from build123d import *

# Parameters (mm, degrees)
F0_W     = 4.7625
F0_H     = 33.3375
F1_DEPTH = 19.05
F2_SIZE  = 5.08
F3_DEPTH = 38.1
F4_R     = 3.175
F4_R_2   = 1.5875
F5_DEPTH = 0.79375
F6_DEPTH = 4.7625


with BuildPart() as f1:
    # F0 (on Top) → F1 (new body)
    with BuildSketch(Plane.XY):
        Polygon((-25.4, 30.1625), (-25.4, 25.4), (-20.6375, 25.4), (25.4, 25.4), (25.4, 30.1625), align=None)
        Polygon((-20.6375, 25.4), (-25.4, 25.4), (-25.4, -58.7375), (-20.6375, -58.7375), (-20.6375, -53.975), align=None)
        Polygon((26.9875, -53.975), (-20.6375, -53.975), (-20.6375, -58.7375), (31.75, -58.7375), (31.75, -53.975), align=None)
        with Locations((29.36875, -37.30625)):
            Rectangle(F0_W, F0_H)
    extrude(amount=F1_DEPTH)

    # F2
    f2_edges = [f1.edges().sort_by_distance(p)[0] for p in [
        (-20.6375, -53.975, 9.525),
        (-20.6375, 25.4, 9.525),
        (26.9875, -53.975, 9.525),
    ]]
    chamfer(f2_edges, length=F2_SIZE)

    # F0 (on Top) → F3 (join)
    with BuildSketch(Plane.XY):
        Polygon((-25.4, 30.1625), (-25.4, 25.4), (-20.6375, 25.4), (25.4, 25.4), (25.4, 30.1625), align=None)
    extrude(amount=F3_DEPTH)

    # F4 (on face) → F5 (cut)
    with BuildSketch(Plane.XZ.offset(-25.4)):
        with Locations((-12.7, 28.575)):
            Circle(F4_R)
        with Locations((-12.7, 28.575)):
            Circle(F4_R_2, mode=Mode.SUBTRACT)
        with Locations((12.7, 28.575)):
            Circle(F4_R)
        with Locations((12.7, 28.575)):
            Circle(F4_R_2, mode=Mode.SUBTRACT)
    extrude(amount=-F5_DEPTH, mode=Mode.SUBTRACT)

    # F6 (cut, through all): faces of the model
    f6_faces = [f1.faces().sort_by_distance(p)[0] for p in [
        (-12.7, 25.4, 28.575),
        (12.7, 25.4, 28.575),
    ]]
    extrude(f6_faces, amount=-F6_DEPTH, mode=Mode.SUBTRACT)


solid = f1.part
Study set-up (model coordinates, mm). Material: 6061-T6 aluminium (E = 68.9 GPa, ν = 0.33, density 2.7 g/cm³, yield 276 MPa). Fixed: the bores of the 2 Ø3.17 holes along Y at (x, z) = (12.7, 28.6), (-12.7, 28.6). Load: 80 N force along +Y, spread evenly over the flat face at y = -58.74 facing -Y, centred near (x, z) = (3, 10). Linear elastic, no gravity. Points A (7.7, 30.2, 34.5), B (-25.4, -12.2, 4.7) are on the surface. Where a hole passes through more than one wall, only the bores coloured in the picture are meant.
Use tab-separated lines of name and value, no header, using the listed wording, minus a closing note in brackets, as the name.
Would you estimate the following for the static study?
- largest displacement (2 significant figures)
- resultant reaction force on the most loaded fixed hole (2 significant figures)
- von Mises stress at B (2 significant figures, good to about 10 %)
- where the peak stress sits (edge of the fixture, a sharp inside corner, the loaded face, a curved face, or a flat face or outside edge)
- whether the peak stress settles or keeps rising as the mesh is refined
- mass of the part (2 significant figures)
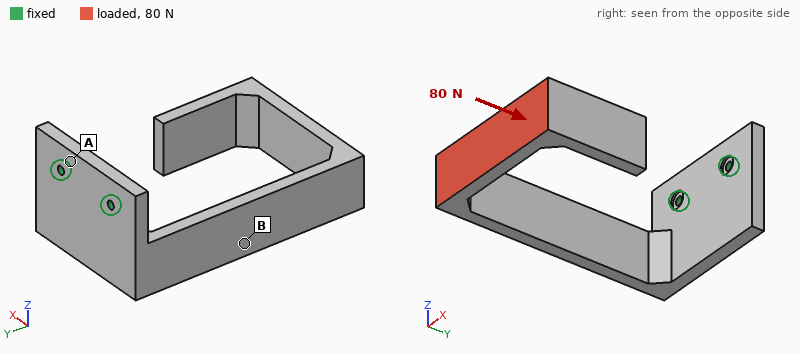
largest displacement	1.1 mm
resultant reaction force on the most loaded fixed hole	46 N
von Mises stress at B	28 MPa
where the peak stress sits	edge of the fixture
whether the peak stress settles or keeps rising as the mesh is refined	keeps rising
mass of the part	68 g
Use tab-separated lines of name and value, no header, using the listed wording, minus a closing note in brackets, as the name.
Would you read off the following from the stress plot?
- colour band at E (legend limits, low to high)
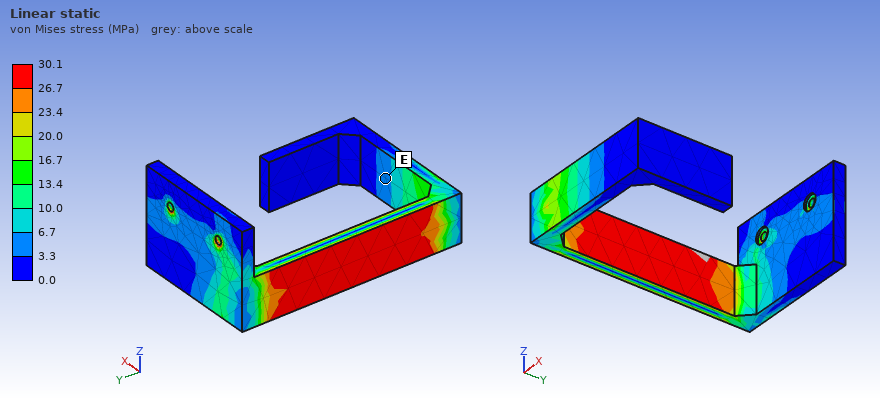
colour band at E	3.3 to 6.7 MPa
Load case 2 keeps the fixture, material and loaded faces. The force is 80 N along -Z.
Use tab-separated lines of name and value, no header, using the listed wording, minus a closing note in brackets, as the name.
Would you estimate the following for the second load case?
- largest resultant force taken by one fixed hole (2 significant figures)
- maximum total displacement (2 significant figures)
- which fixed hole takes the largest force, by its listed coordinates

largest resultant force taken by one fixed hole	52 N
maximum total displacement	1.2 mm
which fixed hole takes the largest force, by its listed coordinates	(12.7, 28.6)
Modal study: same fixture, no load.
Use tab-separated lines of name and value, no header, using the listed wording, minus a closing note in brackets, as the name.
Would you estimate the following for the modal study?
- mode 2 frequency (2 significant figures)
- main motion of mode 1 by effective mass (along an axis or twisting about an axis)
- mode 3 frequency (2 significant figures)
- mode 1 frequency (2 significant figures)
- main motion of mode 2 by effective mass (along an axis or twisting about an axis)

mode 2 frequency	270 Hz
main motion of mode 1 by effective mass	along X
mode 3 frequency	510 Hz
mode 1 frequency	200 Hz
main motion of mode 2 by effective mass	along Z
